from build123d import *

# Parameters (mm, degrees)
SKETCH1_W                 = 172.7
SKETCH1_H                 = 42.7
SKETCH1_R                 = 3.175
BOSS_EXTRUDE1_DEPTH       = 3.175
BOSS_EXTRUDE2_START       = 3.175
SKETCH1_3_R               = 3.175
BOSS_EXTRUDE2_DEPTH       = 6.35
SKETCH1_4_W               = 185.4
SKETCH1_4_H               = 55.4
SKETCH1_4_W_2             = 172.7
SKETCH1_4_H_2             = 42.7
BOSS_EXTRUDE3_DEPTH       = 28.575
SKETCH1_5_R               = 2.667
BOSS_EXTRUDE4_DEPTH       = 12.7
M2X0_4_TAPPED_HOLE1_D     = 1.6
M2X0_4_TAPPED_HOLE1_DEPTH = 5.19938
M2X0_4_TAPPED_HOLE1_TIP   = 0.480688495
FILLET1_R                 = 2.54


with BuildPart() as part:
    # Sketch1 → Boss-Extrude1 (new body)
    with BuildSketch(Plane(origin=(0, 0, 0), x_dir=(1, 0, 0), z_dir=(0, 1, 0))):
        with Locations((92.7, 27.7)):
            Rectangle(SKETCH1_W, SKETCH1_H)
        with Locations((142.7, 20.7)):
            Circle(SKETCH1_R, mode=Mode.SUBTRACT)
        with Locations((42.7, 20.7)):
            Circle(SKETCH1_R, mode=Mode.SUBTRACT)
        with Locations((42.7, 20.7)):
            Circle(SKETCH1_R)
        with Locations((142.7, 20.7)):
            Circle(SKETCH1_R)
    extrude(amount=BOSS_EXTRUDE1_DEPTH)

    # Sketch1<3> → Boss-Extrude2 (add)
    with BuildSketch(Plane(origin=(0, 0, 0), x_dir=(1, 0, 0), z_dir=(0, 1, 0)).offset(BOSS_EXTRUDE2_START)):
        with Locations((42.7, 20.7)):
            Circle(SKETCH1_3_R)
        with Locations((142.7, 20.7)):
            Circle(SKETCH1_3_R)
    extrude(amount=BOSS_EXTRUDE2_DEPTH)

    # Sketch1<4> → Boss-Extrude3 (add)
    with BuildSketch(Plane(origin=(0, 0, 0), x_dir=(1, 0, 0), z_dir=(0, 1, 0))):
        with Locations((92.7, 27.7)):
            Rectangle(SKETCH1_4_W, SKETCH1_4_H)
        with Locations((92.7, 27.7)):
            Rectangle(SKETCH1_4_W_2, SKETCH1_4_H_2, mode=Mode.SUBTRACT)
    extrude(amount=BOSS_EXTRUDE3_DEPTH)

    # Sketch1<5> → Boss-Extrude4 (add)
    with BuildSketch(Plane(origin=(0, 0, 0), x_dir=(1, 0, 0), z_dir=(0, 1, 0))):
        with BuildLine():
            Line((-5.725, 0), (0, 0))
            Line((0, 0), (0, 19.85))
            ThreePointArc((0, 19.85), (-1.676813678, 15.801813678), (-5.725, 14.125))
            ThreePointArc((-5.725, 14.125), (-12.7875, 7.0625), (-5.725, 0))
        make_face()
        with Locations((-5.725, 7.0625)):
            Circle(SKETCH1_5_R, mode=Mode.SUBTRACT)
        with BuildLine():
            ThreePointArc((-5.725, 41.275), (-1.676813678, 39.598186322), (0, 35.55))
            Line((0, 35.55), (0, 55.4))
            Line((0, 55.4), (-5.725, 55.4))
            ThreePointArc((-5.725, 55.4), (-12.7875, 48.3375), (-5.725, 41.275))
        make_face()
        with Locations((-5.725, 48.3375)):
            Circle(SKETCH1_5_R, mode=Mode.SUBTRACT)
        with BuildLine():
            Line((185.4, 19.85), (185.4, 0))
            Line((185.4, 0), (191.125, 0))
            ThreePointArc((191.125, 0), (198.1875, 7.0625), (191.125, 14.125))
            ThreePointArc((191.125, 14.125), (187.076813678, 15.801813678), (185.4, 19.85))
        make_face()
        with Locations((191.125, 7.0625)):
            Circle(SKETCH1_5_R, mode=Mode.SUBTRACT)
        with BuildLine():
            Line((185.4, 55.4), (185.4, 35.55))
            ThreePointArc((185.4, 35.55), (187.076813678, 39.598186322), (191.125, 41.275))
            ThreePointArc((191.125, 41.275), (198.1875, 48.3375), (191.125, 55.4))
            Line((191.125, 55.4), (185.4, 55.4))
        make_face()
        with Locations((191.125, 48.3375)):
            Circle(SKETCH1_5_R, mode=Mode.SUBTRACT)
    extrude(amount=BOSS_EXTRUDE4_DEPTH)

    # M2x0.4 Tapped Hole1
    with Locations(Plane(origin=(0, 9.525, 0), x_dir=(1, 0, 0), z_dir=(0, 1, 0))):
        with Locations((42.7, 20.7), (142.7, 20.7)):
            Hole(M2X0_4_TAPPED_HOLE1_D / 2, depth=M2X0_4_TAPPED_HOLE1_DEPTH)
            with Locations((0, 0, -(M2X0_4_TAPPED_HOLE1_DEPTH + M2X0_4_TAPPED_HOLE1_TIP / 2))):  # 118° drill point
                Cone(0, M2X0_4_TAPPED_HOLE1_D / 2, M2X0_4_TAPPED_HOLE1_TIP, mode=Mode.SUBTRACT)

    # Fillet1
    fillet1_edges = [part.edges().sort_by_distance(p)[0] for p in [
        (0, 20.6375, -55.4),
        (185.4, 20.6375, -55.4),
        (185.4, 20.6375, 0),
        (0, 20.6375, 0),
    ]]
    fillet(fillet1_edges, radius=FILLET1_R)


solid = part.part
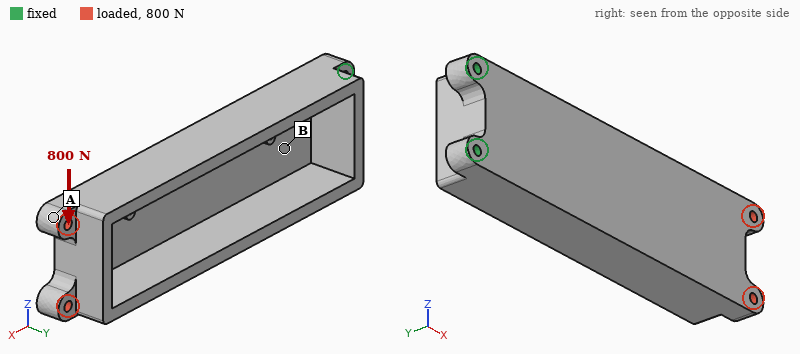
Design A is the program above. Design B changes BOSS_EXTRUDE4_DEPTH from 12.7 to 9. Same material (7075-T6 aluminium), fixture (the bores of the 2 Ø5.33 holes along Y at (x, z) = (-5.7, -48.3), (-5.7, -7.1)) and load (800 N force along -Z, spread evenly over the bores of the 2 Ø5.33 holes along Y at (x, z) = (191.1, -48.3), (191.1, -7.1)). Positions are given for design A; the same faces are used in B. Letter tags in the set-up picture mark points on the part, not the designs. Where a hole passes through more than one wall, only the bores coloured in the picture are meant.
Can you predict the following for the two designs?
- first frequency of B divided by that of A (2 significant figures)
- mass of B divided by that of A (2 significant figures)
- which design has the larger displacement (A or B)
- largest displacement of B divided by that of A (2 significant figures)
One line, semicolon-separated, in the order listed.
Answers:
0.74; 0.98; A; 0.89
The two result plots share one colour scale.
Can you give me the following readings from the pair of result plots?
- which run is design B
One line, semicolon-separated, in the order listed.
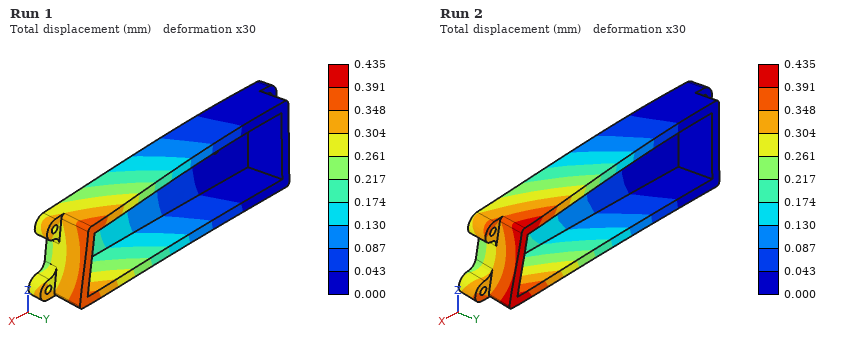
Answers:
Run 1
